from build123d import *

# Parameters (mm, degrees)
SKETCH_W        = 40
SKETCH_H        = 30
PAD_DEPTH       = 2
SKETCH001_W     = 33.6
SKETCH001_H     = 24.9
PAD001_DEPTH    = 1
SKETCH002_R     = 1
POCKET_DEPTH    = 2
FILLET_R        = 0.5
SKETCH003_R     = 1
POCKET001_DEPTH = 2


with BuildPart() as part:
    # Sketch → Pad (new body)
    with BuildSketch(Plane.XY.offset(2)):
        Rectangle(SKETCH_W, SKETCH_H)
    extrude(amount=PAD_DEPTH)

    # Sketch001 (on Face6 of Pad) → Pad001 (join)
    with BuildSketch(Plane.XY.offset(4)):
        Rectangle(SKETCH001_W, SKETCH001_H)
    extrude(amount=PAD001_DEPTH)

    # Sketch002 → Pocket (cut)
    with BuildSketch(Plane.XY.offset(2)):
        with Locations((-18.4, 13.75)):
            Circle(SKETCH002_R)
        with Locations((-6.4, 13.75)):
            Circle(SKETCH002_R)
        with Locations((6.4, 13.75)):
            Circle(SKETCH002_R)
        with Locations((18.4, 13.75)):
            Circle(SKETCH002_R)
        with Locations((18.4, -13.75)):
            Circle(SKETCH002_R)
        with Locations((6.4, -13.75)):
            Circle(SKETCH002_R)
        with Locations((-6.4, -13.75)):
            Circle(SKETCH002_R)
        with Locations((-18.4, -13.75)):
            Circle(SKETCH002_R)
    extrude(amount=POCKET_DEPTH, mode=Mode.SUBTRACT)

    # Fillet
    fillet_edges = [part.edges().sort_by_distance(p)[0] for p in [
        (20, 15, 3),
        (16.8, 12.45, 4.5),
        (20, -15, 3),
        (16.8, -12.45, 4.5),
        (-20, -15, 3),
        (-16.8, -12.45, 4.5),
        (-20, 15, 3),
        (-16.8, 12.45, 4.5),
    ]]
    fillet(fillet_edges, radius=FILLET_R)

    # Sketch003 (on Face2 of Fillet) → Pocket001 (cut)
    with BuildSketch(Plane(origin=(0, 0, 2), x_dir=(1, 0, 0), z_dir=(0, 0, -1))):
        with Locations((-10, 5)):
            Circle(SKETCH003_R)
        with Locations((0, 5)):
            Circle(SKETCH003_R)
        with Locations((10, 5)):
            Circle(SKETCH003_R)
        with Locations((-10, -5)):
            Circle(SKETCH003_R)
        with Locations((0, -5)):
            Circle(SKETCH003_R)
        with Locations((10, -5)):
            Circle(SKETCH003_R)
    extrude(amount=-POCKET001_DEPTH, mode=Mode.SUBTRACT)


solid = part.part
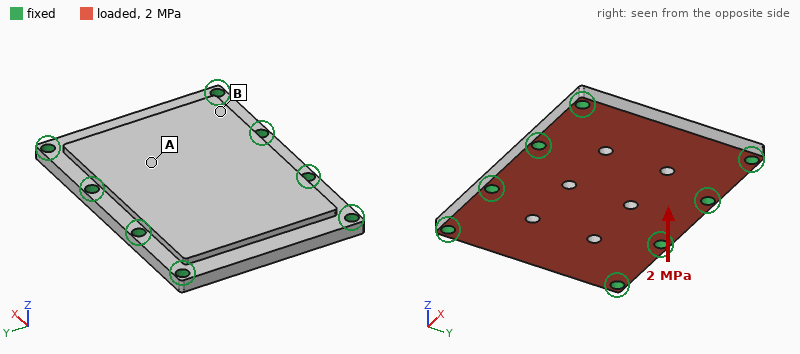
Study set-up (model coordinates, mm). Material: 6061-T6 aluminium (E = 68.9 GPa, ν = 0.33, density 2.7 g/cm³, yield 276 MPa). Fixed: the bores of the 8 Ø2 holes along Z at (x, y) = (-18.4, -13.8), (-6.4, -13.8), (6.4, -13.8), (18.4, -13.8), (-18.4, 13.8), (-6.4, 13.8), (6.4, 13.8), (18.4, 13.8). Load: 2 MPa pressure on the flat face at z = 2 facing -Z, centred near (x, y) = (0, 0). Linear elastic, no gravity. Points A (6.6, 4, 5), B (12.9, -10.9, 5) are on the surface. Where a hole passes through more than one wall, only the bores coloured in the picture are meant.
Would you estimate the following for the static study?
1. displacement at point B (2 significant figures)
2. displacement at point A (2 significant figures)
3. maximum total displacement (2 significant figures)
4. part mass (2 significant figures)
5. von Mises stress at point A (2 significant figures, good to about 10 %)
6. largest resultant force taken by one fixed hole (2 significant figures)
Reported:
13 µm
34 µm
50 µm
8.5 g
56 MPa
430 N
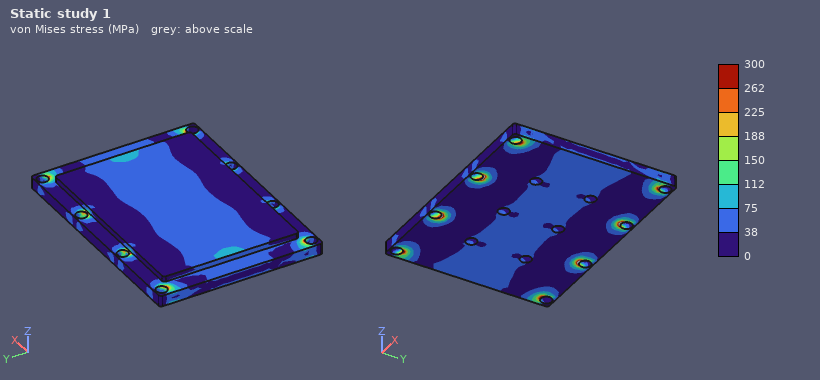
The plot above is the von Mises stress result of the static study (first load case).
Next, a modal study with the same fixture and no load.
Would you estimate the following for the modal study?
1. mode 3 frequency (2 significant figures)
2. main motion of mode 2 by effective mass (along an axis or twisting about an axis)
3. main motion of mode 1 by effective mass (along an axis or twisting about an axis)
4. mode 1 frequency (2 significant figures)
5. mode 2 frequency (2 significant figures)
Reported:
24 kHz
twisting about Y
along Z
14 kHz
17 kHz
